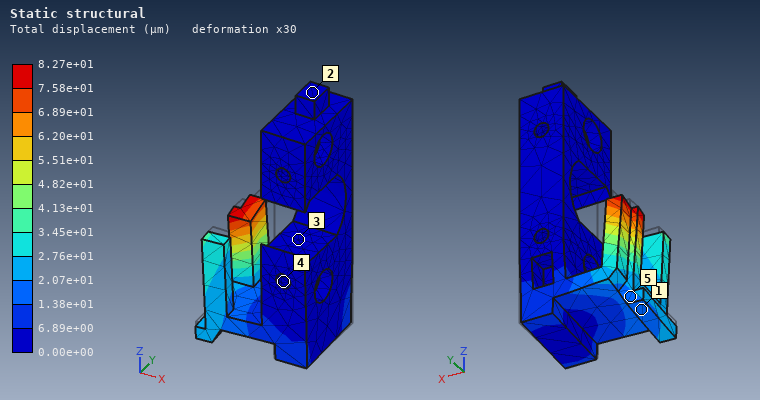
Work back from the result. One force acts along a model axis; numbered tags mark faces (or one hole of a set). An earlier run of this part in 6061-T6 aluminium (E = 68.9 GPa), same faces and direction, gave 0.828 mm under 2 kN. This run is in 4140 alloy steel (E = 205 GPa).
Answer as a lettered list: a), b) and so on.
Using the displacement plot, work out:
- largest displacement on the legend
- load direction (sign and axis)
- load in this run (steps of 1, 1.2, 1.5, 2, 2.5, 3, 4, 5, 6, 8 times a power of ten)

a) 8.27e+01 µm
b) -Y
c) 600 N
